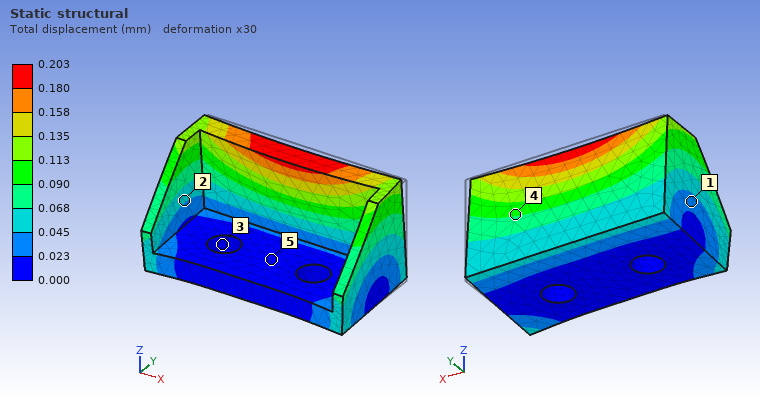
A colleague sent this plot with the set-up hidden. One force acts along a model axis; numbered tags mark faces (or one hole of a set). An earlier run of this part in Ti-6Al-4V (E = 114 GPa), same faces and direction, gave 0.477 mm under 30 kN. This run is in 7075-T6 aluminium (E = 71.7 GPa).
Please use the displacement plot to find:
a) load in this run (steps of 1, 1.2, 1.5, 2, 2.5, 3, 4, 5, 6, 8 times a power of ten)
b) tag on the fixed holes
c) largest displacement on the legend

8 kN
3
0.203 mm
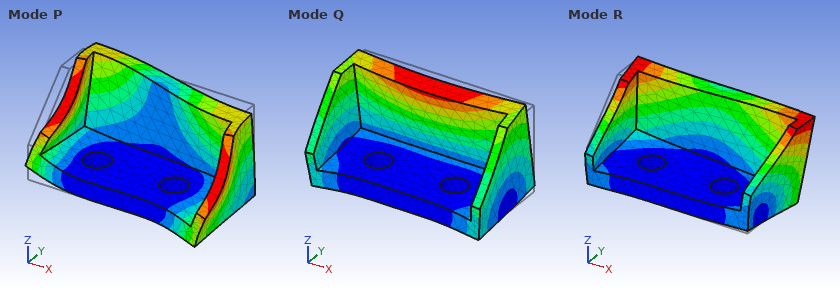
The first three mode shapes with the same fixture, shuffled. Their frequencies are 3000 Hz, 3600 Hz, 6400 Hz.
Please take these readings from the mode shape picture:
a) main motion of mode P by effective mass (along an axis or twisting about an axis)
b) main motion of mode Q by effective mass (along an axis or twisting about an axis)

along X
along Y
